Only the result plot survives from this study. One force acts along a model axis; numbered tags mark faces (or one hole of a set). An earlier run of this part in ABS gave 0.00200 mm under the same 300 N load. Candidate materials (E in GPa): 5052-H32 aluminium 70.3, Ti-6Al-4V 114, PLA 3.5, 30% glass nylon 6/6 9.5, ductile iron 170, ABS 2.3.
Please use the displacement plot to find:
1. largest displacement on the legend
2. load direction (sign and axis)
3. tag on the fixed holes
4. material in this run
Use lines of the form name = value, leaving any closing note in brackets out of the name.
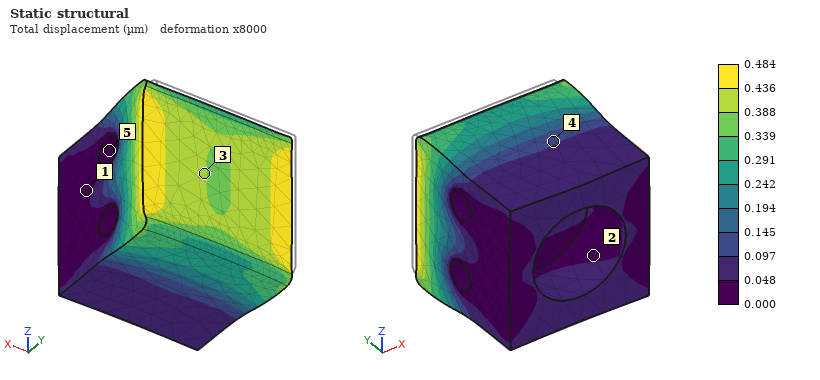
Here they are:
largest displacement on the legend = 0.484 µm
load direction = -Y
tag on the fixed holes = 5
material in this run = 30% glass nylon 6/6
